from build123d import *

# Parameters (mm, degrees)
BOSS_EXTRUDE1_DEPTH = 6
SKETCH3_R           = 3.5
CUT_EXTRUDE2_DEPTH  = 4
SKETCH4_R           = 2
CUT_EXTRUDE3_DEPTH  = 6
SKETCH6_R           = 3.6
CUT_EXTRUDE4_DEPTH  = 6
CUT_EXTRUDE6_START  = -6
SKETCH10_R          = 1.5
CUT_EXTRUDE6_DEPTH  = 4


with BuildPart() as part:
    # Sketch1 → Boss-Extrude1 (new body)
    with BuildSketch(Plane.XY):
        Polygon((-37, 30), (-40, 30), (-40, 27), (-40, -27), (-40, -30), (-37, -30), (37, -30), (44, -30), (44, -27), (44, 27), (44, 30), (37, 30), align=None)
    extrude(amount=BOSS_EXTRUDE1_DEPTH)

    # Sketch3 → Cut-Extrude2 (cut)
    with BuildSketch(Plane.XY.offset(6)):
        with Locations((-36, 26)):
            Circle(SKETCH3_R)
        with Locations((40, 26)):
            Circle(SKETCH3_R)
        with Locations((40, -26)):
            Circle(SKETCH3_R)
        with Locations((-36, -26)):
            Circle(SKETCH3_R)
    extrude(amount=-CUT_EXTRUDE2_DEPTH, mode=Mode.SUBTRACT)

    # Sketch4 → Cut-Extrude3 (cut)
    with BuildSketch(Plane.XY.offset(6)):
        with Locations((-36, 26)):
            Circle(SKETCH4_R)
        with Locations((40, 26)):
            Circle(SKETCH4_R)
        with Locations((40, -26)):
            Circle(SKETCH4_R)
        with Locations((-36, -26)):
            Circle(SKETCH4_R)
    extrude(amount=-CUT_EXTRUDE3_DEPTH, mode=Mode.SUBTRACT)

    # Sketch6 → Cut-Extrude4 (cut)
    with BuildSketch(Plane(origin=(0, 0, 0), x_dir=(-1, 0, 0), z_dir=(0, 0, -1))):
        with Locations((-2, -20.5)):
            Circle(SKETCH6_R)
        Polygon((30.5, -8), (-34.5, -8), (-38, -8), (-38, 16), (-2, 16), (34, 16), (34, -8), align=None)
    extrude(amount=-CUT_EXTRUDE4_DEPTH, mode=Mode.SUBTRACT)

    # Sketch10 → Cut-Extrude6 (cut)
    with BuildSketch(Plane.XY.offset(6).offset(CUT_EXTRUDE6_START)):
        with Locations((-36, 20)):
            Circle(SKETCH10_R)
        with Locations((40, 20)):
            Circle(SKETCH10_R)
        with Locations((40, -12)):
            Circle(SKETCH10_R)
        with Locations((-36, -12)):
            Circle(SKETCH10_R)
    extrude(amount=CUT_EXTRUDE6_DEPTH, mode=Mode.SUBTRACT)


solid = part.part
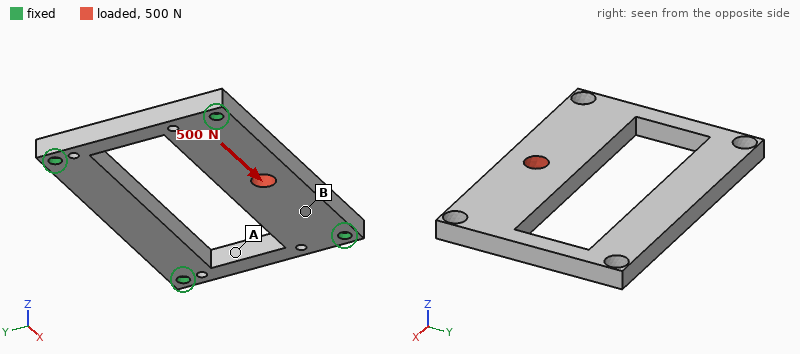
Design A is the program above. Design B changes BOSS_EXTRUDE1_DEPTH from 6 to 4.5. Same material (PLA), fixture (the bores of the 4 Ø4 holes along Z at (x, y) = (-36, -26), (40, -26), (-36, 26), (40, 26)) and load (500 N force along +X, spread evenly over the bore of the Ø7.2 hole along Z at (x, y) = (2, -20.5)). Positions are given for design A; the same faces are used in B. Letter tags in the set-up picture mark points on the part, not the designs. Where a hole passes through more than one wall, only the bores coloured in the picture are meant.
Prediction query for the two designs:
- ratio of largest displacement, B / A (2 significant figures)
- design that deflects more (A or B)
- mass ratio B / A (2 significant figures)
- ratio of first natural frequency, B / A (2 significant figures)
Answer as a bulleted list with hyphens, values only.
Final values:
- 1.1
- B
- 0.75
- 0.83
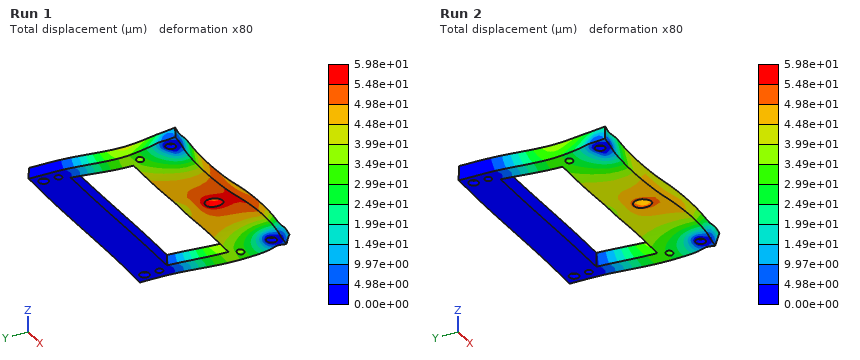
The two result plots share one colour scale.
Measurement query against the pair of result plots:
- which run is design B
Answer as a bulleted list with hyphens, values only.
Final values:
- Run 1
